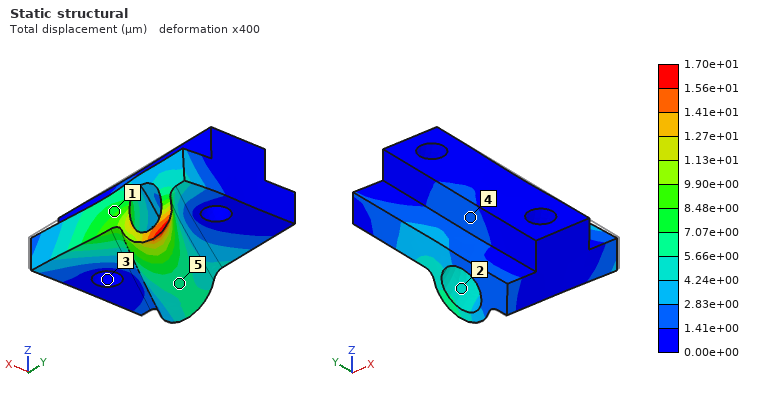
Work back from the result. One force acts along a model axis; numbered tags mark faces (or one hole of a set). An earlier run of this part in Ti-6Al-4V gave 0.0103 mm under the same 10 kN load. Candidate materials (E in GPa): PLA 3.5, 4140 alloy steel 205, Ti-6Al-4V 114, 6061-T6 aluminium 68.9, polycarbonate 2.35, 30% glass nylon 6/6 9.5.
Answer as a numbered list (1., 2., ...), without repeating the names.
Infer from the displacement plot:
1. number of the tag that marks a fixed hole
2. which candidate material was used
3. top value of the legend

1. 3
2. 6061-T6 aluminium
3. 1.70e+01 µm
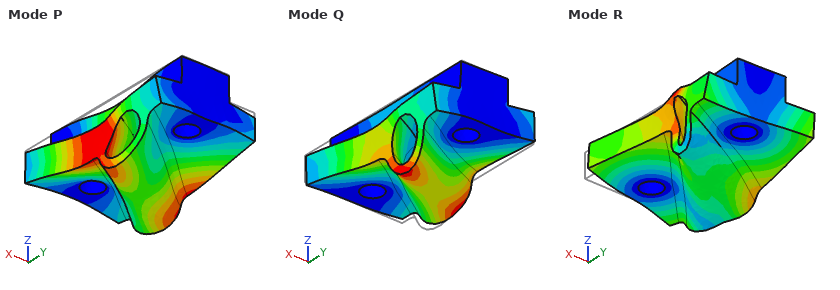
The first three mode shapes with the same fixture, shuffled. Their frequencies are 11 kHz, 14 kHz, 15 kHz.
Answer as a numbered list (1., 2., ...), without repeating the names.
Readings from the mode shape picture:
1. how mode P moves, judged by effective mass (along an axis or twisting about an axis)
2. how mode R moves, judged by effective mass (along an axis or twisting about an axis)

1. along Z
2. along X
